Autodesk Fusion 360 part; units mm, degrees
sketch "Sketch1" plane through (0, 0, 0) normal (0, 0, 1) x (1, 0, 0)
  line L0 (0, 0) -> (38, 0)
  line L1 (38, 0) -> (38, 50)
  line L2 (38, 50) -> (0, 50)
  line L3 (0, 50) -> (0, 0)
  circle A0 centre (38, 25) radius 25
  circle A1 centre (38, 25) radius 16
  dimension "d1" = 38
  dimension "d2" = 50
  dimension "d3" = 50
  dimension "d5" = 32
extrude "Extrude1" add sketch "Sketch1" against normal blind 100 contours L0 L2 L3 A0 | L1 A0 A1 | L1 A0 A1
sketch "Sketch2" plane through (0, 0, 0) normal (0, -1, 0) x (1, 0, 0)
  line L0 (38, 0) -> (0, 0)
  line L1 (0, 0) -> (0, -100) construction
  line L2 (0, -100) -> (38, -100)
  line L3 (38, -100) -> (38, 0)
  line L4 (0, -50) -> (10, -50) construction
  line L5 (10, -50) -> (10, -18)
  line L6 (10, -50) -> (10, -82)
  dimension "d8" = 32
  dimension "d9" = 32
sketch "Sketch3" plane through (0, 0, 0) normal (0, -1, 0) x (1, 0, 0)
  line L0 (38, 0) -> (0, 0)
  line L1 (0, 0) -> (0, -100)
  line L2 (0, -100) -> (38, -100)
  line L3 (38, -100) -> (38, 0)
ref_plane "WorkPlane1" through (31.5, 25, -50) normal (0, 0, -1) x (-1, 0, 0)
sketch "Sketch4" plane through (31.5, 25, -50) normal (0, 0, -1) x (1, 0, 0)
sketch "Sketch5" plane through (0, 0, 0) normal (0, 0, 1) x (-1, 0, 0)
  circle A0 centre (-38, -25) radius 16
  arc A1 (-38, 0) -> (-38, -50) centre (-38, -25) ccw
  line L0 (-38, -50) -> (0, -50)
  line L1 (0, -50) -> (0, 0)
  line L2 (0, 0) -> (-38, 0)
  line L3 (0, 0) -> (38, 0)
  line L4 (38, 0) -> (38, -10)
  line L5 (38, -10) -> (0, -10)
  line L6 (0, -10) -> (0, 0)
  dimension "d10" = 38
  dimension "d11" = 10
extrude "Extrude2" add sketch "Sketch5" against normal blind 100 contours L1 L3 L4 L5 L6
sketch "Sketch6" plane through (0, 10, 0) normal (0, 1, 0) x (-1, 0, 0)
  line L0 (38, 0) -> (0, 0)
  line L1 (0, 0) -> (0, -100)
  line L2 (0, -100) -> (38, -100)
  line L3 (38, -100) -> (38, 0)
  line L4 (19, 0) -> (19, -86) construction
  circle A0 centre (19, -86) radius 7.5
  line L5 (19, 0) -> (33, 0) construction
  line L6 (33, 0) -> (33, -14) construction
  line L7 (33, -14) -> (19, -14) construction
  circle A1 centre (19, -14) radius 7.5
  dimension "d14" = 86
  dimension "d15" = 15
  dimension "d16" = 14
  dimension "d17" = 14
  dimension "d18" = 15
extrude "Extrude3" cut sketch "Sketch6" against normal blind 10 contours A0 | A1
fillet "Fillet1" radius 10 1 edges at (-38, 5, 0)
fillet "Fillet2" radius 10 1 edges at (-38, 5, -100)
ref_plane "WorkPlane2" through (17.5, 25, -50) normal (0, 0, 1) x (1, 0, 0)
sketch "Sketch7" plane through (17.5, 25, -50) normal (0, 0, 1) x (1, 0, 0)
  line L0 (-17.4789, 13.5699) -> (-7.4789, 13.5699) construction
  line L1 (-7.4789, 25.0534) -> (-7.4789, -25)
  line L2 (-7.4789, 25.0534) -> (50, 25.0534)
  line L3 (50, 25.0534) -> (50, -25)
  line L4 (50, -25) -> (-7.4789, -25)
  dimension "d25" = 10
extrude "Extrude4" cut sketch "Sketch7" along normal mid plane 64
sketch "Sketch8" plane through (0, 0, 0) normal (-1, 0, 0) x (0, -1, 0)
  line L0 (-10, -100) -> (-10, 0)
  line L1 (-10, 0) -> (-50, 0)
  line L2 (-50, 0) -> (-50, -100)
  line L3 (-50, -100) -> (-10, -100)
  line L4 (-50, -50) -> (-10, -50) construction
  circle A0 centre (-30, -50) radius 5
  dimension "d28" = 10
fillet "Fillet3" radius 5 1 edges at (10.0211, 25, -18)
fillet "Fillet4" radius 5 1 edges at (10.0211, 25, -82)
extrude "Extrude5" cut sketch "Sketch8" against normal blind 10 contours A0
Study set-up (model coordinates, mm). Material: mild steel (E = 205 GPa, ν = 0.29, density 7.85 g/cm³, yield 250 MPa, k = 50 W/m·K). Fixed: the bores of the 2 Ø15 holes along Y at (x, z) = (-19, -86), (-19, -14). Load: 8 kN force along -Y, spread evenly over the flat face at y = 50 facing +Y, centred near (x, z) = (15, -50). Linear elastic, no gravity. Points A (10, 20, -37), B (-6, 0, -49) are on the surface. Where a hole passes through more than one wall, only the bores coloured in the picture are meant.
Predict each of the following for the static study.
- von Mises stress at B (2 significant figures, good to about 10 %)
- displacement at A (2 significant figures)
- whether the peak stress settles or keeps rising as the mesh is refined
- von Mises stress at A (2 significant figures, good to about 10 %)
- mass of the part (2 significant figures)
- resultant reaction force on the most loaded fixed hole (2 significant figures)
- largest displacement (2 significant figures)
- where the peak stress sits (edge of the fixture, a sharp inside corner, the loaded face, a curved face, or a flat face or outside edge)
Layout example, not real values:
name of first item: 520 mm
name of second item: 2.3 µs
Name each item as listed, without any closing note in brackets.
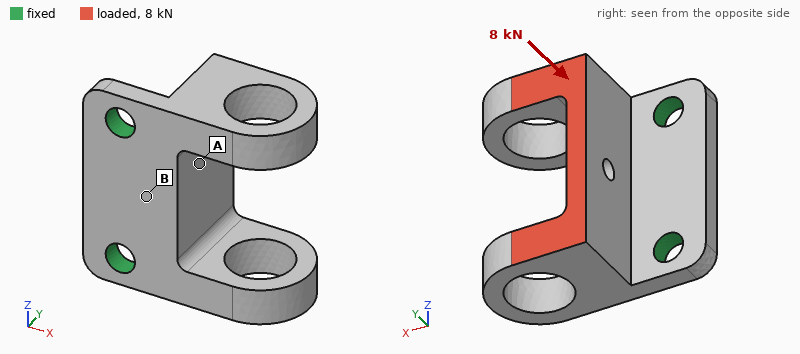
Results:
von Mises stress at B: 48 MPa
displacement at A: 0.048 mm
whether the peak stress settles or keeps rising as the mesh is refined: keeps rising
von Mises stress at A: 21 MPa
mass of the part: 1.1 kg
resultant reaction force on the most loaded fixed hole: 4.0 kN
largest displacement: 0.17 mm
where the peak stress sits: edge of the fixture
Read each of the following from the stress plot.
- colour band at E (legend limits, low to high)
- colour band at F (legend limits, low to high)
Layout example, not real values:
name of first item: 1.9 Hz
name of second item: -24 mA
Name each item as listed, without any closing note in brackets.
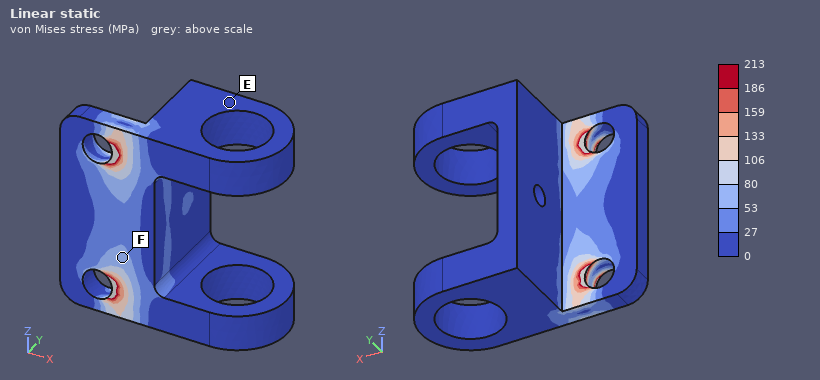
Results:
colour band at E: 0 to 27 MPa
colour band at F: 53 to 80 MPa
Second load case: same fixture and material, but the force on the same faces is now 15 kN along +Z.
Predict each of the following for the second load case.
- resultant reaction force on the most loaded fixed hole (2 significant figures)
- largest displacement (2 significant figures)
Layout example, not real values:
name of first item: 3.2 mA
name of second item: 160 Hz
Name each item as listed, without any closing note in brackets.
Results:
resultant reaction force on the most loaded fixed hole: 13 kN
largest displacement: 88 µm
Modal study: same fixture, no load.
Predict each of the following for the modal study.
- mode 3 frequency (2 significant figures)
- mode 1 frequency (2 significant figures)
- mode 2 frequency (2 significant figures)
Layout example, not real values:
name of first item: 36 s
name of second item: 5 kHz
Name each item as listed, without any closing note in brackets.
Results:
mode 3 frequency: 3100 Hz
mode 1 frequency: 1200 Hz
mode 2 frequency: 1700 Hz
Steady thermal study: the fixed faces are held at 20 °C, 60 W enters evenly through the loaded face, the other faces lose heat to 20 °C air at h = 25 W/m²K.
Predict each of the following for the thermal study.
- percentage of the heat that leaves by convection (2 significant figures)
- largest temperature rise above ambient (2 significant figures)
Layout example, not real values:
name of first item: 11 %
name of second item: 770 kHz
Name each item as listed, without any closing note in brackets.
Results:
percentage of the heat that leaves by convection: 33 %
largest temperature rise above ambient: 48 K
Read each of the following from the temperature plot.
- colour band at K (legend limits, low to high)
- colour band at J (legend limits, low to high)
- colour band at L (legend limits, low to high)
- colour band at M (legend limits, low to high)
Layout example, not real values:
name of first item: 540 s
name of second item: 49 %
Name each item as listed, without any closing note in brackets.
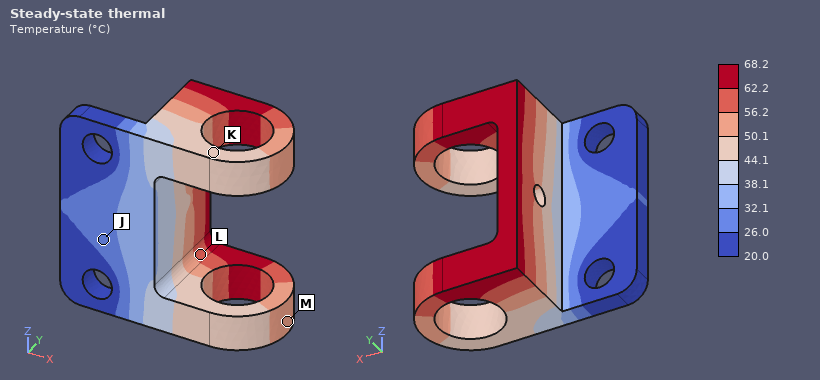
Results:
colour band at K: 44.1 to 50.1 °C
colour band at J: 26.0 to 32.1 °C
colour band at L: 56.2 to 62.2 °C
colour band at M: 50.1 to 56.2 °C
